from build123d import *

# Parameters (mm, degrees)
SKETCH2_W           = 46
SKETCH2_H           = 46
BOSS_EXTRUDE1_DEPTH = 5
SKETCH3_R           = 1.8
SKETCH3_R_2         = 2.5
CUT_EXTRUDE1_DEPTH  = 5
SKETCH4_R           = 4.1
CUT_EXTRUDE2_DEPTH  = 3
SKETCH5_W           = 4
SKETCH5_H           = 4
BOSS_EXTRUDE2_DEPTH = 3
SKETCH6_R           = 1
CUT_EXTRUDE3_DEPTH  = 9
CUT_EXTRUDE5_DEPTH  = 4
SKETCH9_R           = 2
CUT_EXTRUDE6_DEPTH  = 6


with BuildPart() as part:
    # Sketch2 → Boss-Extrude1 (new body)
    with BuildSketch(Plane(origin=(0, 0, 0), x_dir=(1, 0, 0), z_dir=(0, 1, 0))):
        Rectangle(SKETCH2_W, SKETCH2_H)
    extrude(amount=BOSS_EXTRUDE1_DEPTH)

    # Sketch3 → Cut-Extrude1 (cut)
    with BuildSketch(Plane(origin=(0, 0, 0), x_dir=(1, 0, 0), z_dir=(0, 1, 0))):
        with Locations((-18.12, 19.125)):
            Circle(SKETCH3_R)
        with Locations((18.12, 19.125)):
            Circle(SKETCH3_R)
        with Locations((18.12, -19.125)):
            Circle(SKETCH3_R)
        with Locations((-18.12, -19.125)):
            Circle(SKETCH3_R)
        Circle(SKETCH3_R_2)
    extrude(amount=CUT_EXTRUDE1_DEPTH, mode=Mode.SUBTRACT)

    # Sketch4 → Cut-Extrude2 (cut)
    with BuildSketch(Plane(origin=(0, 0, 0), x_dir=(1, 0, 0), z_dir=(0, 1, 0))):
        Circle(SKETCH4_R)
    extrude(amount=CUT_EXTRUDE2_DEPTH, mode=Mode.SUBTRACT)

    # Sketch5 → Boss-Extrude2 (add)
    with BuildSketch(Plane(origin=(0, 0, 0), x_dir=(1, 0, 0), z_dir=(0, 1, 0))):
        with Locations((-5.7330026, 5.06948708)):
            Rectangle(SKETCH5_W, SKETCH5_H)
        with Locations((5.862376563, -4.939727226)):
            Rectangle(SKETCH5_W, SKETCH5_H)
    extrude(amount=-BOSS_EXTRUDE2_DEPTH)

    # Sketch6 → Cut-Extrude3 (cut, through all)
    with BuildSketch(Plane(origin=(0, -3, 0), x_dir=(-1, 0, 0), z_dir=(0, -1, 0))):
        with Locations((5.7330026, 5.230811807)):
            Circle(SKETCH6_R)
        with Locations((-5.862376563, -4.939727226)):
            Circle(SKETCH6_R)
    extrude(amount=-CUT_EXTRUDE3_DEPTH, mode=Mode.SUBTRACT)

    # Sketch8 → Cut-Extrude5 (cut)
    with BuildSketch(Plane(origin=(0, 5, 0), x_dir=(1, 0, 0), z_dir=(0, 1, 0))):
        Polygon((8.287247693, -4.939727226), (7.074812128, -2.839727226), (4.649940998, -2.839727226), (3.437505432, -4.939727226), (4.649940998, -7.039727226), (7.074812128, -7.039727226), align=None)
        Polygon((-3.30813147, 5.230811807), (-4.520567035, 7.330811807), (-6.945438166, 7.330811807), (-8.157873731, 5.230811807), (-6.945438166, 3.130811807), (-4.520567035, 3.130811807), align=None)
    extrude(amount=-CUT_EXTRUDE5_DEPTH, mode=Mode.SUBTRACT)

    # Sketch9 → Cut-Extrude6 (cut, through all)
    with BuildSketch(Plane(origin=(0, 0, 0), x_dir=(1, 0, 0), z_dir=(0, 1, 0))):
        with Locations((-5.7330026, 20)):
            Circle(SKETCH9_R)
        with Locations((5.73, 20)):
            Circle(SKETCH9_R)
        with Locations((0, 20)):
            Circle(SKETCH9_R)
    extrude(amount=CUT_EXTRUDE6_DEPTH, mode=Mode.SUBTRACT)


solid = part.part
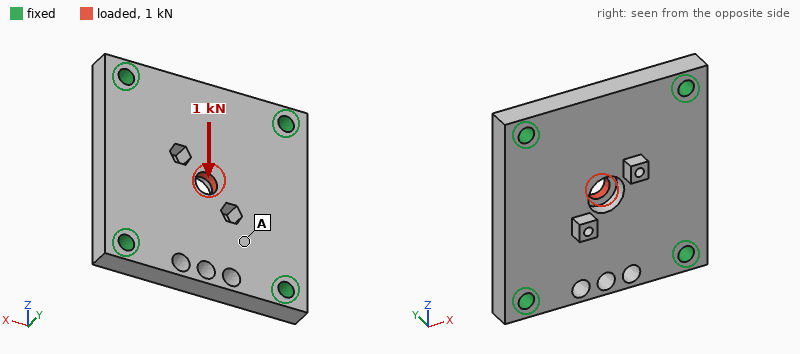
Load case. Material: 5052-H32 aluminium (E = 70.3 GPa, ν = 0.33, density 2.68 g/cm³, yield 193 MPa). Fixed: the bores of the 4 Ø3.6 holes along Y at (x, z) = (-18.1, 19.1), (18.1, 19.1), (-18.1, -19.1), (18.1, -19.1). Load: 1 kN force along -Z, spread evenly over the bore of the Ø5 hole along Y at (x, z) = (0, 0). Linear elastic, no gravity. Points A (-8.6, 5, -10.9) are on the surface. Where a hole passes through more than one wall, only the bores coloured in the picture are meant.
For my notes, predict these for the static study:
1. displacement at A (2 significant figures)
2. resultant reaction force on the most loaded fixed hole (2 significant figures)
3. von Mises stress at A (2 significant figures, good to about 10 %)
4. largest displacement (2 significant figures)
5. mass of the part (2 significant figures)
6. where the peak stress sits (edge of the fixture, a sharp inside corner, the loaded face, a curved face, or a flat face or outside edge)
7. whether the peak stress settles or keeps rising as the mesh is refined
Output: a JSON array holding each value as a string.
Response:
["1.3 µm", "290 N", "5.3 MPa", "4.3 µm", "27 g", "a sharp inside corner", "keeps rising"]
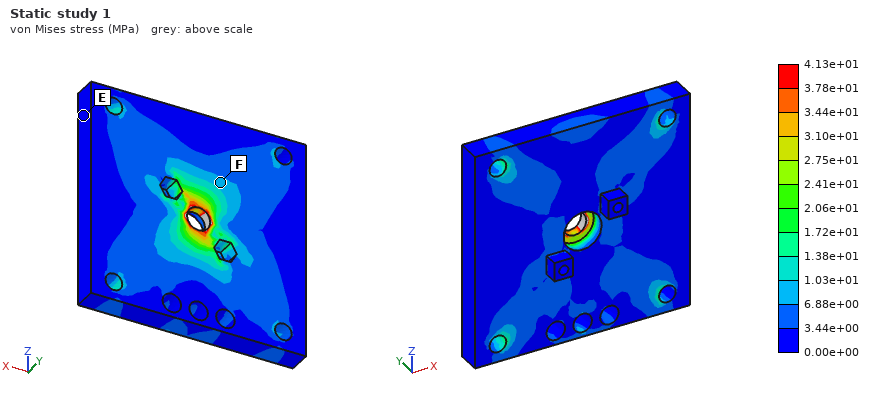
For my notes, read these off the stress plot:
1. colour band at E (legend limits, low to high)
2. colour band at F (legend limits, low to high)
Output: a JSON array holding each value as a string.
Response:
["0.00e+00 to 3.44e+00 MPa", "6.88e+00 to 1.03e+01 MPa"]
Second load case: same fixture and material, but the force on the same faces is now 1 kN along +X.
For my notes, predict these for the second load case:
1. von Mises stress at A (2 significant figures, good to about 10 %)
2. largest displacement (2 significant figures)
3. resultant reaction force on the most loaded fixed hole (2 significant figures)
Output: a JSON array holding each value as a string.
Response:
["5.8 MPa", "4.6 µm", "290 N"]
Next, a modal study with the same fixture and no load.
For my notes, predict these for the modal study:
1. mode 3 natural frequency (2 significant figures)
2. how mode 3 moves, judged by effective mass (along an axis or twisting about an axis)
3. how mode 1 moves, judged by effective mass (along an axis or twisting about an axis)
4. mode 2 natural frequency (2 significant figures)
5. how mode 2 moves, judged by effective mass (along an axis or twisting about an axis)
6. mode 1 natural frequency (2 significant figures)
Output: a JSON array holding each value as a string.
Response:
["20 kHz", "twisting about X", "along Y", "18 kHz", "twisting about Z", "12 kHz"]
